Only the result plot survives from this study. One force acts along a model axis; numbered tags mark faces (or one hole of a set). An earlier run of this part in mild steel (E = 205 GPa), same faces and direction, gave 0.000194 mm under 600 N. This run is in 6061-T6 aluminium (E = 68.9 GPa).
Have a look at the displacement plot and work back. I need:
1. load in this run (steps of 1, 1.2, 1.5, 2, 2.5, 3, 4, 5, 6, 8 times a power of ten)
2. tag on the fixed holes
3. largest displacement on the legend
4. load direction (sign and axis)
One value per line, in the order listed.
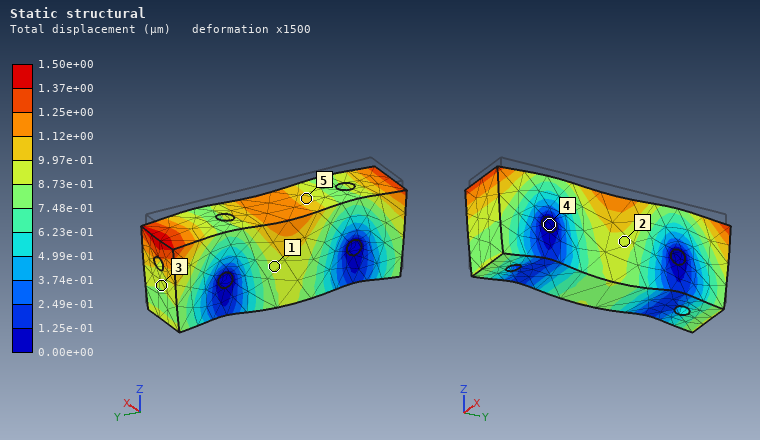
1.5 kN
4
1.50e+00 µm
-Z
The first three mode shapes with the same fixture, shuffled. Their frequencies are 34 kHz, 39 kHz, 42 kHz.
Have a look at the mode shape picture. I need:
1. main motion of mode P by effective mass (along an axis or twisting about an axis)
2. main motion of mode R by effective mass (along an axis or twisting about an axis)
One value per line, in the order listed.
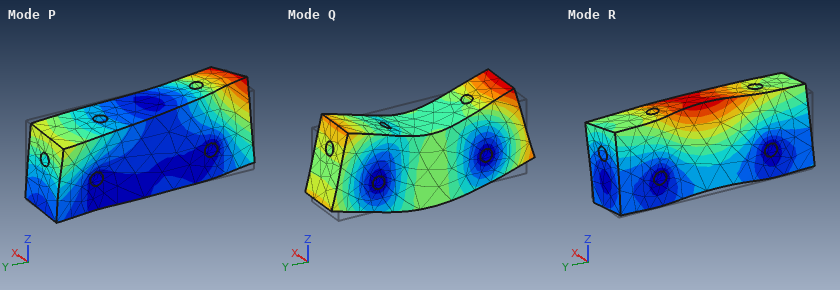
twisting about Z
along X
